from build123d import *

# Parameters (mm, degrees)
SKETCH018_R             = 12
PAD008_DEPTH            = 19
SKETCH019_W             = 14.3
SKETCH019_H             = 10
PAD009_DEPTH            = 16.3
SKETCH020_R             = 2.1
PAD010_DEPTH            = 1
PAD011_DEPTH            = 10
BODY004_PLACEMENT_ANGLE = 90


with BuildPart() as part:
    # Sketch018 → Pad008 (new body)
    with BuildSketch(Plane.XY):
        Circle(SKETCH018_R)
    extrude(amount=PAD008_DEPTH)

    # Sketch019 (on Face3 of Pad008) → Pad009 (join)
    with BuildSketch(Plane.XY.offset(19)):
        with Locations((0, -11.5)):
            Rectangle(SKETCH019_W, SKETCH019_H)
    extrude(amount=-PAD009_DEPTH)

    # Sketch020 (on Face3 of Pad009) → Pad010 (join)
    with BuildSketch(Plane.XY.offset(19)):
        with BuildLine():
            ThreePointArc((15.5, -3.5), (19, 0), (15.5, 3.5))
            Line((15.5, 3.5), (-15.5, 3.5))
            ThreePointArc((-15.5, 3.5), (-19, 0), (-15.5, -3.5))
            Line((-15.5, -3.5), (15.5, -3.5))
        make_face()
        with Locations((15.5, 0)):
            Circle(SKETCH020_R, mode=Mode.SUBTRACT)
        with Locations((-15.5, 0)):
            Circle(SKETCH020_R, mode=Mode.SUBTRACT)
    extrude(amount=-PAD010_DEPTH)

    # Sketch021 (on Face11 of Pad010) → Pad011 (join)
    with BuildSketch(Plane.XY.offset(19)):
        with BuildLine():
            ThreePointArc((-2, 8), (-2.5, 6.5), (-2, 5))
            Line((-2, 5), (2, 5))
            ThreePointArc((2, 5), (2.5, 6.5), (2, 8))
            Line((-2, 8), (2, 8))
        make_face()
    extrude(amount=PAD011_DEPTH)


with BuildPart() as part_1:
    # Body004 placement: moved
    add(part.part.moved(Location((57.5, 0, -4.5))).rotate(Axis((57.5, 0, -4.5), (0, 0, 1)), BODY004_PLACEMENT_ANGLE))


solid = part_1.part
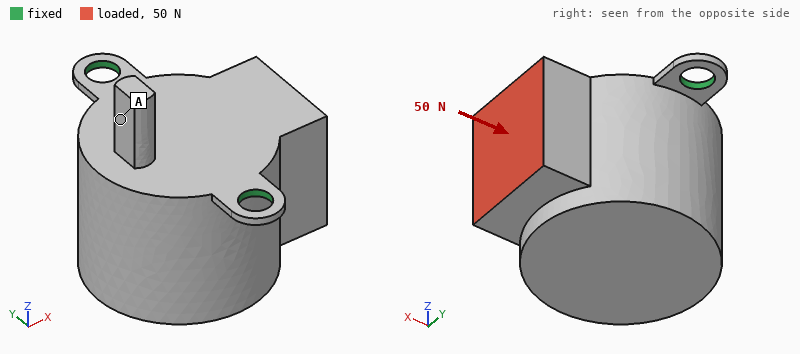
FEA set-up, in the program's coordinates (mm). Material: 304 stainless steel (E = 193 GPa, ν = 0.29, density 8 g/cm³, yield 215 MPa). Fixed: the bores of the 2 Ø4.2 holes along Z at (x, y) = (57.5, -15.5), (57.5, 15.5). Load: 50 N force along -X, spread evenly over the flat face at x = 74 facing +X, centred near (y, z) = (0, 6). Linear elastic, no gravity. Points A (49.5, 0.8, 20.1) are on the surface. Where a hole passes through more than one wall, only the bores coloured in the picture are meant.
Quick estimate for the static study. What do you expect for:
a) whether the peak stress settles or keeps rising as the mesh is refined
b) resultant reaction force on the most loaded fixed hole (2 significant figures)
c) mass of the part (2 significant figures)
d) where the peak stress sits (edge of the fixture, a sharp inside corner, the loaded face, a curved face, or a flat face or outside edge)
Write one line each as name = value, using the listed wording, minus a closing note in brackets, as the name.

whether the peak stress settles or keeps rising as the mesh is refined = keeps rising
resultant reaction force on the most loaded fixed hole = 25 N
mass of the part = 80 g
where the peak stress sits = edge of the fixture
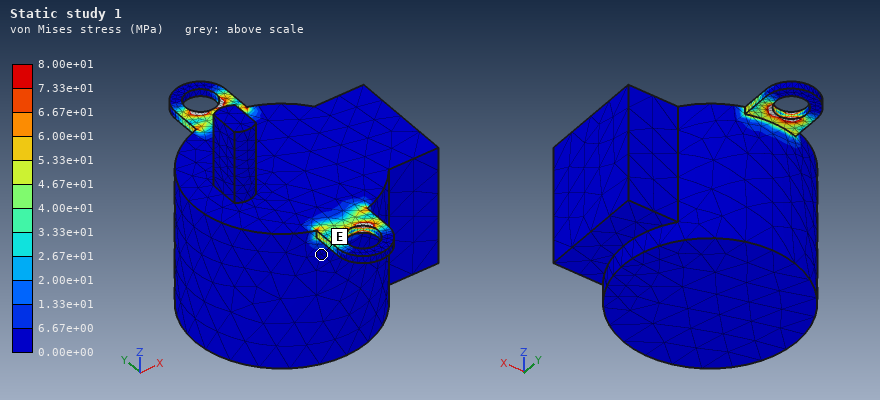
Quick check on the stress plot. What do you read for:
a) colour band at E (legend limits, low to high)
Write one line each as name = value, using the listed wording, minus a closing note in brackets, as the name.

colour band at E = 0.00e+00 to 6.67e+00 MPa
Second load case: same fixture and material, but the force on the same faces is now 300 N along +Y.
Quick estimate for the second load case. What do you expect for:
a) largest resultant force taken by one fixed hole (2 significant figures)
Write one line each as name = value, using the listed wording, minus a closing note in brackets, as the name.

largest resultant force taken by one fixed hole = 250 N
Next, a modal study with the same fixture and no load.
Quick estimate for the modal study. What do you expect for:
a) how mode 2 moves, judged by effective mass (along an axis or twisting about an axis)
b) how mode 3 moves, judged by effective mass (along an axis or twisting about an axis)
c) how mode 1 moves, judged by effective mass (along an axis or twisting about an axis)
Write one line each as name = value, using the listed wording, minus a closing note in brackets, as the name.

how mode 2 moves, judged by effective mass = along Z
how mode 3 moves, judged by effective mass = along Y
how mode 1 moves, judged by effective mass = along X
